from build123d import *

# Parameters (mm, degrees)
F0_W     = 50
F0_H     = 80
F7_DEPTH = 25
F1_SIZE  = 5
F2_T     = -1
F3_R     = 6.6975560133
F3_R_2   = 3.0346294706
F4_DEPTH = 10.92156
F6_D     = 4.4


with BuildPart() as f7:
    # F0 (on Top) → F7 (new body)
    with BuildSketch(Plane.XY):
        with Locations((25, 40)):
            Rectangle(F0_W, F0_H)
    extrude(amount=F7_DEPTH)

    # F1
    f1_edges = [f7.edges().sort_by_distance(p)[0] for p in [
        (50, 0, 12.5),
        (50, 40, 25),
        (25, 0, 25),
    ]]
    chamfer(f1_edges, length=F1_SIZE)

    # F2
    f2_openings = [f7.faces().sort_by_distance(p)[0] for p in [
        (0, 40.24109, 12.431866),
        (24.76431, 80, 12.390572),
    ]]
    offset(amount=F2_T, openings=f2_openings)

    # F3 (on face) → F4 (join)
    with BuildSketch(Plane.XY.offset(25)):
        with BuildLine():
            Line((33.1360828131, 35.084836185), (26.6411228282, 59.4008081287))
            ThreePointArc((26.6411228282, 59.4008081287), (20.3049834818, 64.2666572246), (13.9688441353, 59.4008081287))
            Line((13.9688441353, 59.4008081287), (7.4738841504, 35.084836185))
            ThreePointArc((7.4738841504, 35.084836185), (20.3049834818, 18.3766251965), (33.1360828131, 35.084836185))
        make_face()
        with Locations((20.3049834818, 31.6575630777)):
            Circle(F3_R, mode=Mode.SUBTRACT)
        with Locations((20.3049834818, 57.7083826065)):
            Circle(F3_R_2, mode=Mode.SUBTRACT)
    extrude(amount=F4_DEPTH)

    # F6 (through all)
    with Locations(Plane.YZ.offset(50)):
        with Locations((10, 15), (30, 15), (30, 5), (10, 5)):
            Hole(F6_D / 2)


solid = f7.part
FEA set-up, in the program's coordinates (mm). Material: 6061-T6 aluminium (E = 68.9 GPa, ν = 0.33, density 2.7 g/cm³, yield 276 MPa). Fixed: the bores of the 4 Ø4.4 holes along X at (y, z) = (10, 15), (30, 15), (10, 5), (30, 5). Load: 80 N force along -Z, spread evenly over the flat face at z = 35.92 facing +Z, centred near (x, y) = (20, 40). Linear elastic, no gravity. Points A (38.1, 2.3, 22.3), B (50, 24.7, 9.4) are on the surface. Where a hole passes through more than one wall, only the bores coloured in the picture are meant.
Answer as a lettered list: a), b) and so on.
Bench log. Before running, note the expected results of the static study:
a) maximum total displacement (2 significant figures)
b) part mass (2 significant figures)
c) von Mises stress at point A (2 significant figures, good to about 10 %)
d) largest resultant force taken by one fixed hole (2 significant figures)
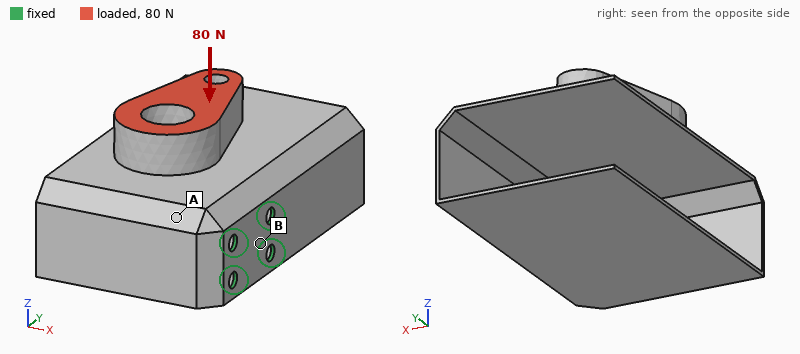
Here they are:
a) 1.1 mm
b) 49 g
c) 16 MPa
d) 160 N
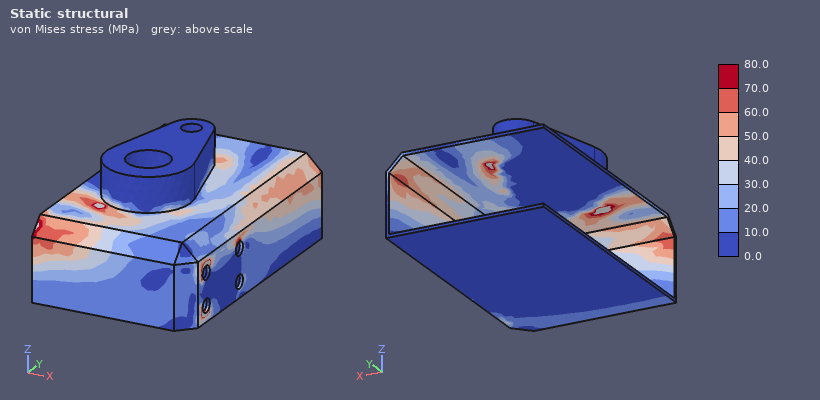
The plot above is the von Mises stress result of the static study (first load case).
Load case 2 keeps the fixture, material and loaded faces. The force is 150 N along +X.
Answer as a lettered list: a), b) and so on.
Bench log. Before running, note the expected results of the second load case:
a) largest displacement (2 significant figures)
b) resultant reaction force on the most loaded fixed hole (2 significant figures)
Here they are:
a) 1.1 mm
b) 220 N
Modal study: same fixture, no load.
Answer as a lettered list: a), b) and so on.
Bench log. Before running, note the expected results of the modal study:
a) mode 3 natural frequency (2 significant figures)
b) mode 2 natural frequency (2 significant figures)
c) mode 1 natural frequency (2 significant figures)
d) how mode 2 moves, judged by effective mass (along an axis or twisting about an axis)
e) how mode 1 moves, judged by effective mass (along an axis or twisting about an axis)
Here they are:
a) 680 Hz
b) 410 Hz
c) 340 Hz
d) along Z
e) along Z
